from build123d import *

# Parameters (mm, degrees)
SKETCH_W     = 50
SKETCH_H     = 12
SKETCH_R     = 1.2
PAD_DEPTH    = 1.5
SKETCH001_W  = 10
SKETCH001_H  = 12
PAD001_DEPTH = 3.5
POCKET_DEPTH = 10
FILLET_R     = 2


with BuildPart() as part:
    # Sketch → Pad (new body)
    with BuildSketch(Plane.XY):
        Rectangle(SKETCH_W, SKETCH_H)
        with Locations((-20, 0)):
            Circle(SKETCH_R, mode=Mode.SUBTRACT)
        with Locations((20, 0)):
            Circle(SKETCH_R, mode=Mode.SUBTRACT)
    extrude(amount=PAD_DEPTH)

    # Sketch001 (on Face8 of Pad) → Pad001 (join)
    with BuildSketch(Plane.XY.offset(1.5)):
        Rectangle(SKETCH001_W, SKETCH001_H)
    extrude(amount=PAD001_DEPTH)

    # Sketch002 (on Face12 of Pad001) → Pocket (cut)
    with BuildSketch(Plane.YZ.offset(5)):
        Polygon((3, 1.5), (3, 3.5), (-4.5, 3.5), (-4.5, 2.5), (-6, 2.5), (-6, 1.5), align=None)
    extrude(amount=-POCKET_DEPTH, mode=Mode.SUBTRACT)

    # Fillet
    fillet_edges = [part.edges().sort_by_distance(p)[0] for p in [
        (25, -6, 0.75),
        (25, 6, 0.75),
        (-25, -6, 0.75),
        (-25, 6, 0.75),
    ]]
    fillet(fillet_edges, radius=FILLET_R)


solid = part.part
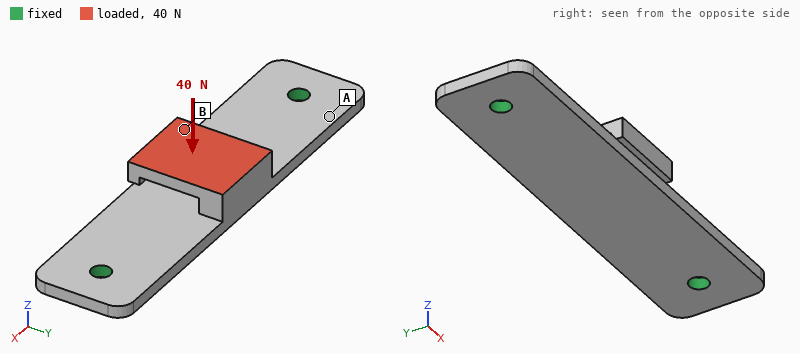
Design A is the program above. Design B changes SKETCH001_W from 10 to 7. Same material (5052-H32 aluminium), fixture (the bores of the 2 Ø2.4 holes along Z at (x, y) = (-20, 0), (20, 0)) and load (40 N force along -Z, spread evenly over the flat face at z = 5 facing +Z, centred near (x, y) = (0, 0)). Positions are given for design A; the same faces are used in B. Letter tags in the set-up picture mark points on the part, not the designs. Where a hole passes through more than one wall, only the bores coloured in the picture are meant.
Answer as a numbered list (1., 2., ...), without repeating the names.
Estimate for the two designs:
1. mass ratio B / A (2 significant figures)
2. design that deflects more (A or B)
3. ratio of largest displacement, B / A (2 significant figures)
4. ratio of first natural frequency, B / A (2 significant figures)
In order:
1. 0.93
2. B
3. 1.2
4. 1.0
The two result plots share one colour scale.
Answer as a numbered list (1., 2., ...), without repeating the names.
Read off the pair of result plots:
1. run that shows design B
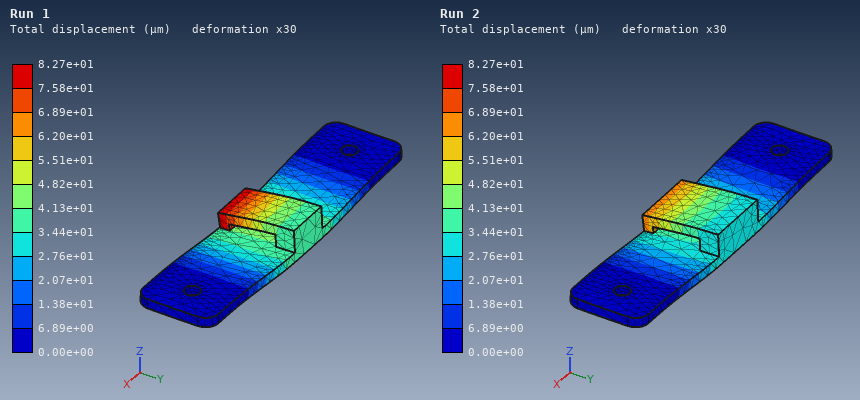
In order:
1. Run 1
